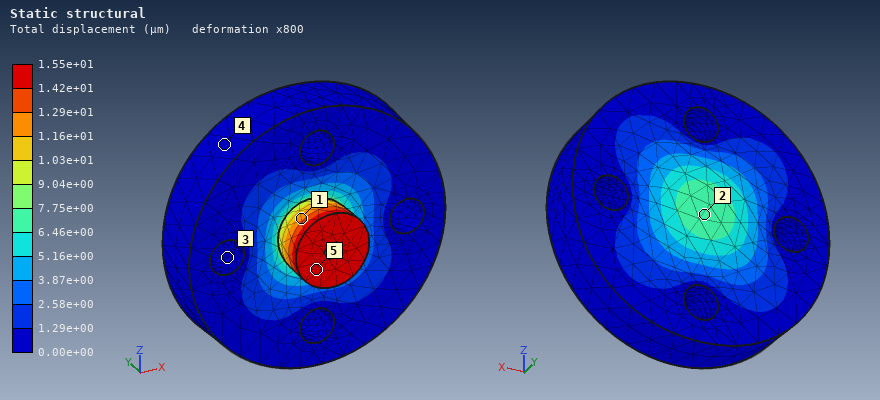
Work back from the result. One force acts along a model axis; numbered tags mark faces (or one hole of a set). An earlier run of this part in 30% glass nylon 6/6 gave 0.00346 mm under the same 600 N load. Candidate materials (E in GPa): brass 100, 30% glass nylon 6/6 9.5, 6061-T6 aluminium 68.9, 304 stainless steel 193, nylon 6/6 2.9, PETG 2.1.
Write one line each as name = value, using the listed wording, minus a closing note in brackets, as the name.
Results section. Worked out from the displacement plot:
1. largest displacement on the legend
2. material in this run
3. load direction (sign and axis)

largest displacement on the legend = 1.55e+01 µm
material in this run = PETG
load direction = +Y
